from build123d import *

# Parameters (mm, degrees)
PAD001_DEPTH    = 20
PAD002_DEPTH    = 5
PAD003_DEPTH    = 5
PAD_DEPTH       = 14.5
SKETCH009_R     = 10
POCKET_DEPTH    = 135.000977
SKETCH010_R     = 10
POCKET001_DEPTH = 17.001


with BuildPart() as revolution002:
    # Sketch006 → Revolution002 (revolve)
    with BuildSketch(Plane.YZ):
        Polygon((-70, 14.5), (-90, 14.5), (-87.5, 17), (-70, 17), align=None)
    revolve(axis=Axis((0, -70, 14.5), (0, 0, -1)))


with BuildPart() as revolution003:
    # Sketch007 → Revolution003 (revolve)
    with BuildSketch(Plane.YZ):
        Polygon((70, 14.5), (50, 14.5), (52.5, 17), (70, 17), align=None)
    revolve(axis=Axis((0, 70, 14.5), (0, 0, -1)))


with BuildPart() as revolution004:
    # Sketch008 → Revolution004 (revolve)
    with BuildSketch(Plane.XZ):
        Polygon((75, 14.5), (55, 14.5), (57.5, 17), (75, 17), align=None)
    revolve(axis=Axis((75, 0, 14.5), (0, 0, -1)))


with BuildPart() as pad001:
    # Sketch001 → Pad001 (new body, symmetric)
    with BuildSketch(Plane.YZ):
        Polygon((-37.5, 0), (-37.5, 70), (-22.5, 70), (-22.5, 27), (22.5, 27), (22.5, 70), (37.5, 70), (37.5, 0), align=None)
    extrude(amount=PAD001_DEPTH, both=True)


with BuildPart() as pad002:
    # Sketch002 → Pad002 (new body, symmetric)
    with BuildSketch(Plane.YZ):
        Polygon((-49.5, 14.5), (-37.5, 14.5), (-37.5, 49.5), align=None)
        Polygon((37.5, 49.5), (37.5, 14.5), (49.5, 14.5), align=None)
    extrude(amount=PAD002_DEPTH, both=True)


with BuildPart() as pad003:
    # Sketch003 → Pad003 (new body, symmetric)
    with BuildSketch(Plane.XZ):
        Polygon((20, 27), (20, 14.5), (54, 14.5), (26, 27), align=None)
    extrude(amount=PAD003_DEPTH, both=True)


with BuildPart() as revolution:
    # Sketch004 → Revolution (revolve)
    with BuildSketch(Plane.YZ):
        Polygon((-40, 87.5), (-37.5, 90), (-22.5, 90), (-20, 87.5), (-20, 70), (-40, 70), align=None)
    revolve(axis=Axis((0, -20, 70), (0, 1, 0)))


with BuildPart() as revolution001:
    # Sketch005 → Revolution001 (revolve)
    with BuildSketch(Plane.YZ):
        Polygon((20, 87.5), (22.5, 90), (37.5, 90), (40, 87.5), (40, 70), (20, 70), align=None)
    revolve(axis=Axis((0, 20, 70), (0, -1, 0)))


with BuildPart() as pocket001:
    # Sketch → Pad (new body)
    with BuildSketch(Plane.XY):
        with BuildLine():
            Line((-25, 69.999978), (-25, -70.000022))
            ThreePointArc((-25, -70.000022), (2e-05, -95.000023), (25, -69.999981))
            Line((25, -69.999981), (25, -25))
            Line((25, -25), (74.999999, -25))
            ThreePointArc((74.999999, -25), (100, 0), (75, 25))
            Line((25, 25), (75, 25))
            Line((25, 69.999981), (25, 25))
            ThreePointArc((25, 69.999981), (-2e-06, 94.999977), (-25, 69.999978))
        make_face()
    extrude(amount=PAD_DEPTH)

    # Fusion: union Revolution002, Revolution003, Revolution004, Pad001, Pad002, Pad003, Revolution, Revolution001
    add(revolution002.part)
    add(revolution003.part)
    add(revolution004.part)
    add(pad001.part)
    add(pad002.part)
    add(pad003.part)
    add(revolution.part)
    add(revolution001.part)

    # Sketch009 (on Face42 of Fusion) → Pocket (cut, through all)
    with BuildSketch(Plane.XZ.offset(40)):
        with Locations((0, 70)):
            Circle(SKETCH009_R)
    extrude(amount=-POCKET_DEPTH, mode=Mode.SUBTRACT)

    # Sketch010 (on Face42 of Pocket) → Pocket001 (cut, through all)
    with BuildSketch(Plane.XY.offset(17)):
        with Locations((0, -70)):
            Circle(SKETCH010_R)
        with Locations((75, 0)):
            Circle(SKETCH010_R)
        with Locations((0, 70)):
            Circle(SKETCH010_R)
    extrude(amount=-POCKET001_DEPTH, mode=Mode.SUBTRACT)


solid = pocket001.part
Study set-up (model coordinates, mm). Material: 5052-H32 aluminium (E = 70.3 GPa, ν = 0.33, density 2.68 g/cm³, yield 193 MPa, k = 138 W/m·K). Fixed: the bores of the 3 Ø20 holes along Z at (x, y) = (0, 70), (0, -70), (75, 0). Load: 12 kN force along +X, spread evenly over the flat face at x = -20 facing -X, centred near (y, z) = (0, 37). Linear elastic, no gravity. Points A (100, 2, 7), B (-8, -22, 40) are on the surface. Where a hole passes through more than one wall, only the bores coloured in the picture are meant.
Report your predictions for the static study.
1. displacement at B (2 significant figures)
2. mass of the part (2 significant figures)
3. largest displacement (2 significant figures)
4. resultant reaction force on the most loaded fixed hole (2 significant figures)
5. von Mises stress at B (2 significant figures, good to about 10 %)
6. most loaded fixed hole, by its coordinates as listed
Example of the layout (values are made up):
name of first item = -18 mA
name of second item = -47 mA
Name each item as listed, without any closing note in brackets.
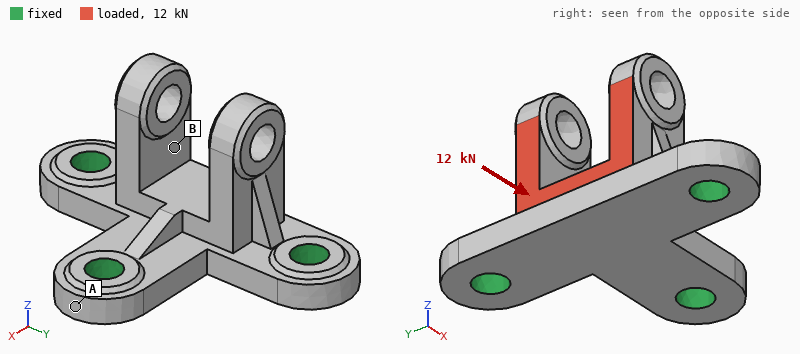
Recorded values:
displacement at B = 0.066 mm
mass of the part = 770 g
largest displacement = 0.15 mm
resultant reaction force on the most loaded fixed hole = 8.1 kN
von Mises stress at B = 12 MPa
most loaded fixed hole, by its coordinates as listed = (75, 0)
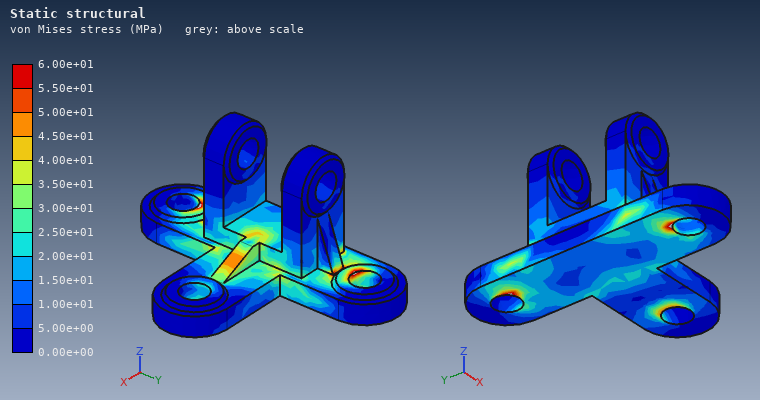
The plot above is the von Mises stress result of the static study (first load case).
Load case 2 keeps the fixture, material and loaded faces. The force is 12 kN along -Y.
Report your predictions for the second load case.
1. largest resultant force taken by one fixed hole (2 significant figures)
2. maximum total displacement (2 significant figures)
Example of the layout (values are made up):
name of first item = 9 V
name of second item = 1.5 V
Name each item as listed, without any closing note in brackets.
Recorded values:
largest resultant force taken by one fixed hole = 7.0 kN
maximum total displacement = 0.12 mm
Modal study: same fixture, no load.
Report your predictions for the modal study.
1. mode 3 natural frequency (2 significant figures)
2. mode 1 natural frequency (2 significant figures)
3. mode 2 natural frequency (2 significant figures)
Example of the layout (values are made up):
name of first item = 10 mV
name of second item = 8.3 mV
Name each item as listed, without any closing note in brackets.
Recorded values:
mode 3 natural frequency = 3100 Hz
mode 1 natural frequency = 2600 Hz
mode 2 natural frequency = 3100 Hz
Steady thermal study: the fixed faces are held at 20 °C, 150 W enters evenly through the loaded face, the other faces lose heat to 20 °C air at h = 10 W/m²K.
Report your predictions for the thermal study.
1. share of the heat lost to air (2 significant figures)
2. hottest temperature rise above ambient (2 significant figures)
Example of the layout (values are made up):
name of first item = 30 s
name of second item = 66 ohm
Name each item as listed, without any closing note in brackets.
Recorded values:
share of the heat lost to air = 4.8 %
hottest temperature rise above ambient = 38 K
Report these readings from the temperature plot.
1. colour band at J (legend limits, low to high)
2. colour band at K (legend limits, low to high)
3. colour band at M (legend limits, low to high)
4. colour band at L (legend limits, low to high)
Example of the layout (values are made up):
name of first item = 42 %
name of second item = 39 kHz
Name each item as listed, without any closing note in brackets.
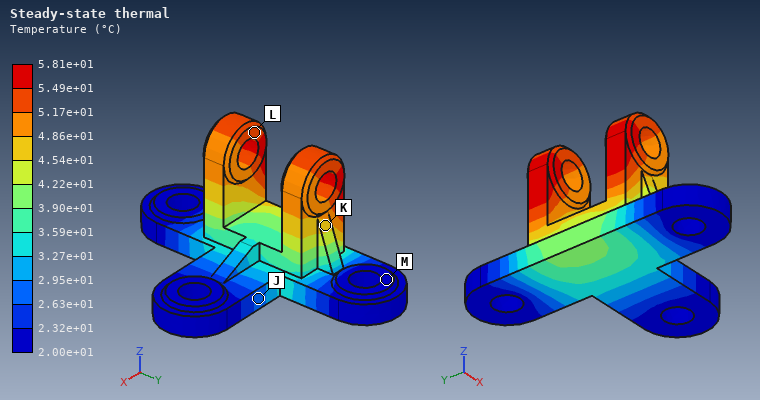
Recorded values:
colour band at J = 2.63e+01 to 2.95e+01 °C
colour band at K = 4.54e+01 to 4.86e+01 °C
colour band at M = 2.00e+01 to 2.32e+01 °C
colour band at L = 5.17e+01 to 5.49e+01 °C
